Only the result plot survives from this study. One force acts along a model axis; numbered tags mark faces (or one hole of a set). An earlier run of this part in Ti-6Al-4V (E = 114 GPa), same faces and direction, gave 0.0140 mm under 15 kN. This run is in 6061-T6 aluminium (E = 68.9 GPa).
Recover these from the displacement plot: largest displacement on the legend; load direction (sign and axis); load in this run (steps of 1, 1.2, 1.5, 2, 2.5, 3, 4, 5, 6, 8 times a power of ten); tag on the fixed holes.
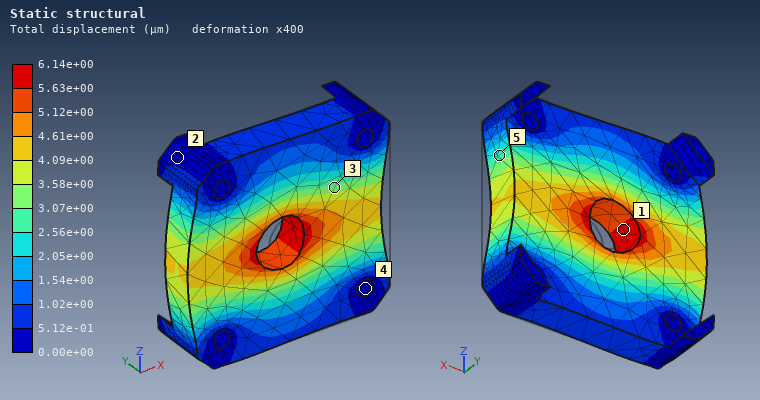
6.14e+00 µm
-X
4 kN
4
